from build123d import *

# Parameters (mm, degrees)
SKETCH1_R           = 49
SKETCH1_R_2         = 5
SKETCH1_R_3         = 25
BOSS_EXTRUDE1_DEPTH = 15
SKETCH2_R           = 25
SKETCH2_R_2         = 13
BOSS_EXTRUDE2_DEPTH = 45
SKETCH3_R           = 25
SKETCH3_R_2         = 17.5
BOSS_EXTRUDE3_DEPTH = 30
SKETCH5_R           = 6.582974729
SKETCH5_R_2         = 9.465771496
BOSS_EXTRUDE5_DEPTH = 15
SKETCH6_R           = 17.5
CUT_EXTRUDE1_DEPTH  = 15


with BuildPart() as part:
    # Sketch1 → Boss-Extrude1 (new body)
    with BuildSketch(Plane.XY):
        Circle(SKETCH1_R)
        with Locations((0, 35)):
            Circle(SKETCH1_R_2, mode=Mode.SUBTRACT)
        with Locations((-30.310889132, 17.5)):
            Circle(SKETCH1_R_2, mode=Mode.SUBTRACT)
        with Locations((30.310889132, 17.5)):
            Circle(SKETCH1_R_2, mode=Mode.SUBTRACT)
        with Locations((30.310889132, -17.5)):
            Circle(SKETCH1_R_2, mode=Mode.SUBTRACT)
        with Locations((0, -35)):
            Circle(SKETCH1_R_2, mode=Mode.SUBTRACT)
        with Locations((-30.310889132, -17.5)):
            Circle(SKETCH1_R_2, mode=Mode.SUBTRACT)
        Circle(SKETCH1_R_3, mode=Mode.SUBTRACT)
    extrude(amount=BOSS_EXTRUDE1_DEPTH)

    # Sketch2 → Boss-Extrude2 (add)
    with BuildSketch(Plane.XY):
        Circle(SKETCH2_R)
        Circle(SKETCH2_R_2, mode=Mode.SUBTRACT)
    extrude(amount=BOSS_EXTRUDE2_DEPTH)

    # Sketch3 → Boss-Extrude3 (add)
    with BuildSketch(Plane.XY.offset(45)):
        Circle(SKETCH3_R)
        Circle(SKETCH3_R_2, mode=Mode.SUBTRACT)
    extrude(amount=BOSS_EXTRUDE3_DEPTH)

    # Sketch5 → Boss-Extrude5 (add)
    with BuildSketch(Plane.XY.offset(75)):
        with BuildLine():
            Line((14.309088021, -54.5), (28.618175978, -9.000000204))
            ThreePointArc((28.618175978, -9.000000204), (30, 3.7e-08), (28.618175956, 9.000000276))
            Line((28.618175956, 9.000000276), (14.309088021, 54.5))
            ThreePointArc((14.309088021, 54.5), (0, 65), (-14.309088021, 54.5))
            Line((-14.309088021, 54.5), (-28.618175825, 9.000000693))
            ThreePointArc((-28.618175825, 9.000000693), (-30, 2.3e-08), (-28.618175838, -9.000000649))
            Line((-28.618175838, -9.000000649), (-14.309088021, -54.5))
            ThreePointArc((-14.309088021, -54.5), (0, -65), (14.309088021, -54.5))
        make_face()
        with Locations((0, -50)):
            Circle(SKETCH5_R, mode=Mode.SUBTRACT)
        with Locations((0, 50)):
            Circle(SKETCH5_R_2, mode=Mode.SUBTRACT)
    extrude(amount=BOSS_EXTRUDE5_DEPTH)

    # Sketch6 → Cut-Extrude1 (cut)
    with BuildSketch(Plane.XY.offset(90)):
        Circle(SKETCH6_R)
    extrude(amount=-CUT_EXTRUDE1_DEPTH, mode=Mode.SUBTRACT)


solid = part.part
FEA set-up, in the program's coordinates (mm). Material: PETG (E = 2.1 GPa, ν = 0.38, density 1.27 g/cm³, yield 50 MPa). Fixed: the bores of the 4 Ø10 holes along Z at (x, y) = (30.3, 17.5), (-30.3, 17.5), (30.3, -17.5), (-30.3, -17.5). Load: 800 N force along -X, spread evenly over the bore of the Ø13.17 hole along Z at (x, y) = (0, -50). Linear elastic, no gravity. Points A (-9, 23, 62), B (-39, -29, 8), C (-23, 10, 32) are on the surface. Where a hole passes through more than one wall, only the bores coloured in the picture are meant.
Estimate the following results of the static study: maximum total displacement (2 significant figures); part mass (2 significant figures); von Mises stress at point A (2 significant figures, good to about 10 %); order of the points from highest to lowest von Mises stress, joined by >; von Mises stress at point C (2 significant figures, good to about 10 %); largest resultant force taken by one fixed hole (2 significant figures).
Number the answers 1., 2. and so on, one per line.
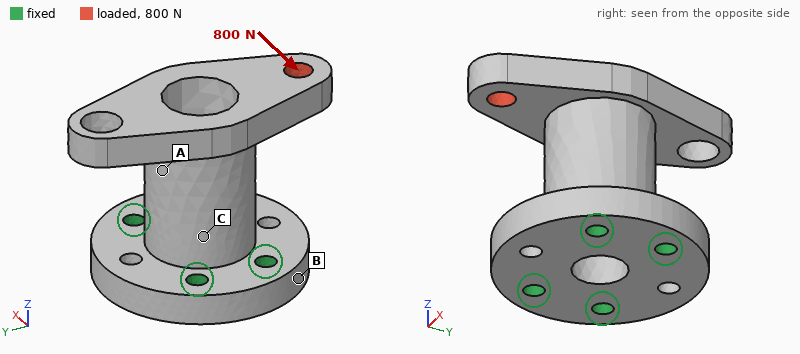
1. 1.0 mm
2. 290 g
3. 1.6 MPa
4. C > A > B
5. 4.3 MPa
6. 710 N
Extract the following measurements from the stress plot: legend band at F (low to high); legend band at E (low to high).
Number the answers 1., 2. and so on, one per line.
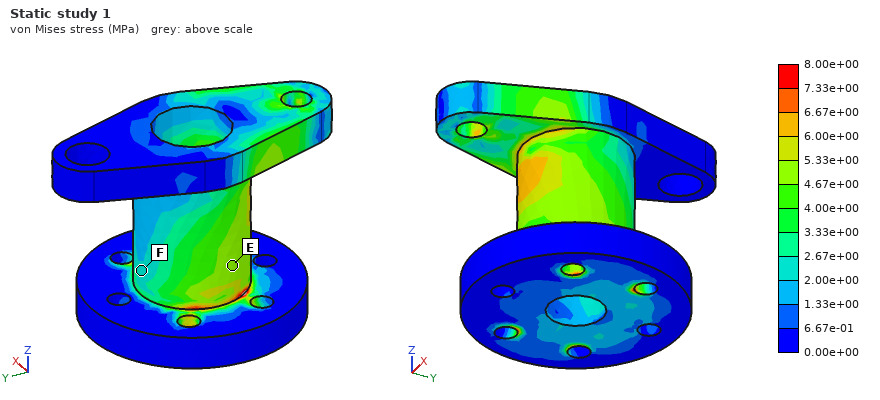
1. 2.00e+00 to 2.67e+00 MPa
2. 4.67e+00 to 5.33e+00 MPa
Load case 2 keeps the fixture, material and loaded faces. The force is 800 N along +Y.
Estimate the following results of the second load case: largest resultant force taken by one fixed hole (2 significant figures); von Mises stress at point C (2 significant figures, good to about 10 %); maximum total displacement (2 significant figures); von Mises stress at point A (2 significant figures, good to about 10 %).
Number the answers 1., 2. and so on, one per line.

1. 770 N
2. 2.2 MPa
3. 0.77 mm
4. 1.7 MPa
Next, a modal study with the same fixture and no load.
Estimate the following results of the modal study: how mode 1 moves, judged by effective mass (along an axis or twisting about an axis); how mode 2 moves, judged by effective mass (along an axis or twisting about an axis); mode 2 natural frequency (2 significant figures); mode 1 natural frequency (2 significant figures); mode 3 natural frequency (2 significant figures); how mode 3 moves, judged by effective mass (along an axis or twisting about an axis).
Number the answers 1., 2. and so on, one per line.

1. along Y
2. along X
3. 760 Hz
4. 600 Hz
5. 1100 Hz
6. twisting about Z
